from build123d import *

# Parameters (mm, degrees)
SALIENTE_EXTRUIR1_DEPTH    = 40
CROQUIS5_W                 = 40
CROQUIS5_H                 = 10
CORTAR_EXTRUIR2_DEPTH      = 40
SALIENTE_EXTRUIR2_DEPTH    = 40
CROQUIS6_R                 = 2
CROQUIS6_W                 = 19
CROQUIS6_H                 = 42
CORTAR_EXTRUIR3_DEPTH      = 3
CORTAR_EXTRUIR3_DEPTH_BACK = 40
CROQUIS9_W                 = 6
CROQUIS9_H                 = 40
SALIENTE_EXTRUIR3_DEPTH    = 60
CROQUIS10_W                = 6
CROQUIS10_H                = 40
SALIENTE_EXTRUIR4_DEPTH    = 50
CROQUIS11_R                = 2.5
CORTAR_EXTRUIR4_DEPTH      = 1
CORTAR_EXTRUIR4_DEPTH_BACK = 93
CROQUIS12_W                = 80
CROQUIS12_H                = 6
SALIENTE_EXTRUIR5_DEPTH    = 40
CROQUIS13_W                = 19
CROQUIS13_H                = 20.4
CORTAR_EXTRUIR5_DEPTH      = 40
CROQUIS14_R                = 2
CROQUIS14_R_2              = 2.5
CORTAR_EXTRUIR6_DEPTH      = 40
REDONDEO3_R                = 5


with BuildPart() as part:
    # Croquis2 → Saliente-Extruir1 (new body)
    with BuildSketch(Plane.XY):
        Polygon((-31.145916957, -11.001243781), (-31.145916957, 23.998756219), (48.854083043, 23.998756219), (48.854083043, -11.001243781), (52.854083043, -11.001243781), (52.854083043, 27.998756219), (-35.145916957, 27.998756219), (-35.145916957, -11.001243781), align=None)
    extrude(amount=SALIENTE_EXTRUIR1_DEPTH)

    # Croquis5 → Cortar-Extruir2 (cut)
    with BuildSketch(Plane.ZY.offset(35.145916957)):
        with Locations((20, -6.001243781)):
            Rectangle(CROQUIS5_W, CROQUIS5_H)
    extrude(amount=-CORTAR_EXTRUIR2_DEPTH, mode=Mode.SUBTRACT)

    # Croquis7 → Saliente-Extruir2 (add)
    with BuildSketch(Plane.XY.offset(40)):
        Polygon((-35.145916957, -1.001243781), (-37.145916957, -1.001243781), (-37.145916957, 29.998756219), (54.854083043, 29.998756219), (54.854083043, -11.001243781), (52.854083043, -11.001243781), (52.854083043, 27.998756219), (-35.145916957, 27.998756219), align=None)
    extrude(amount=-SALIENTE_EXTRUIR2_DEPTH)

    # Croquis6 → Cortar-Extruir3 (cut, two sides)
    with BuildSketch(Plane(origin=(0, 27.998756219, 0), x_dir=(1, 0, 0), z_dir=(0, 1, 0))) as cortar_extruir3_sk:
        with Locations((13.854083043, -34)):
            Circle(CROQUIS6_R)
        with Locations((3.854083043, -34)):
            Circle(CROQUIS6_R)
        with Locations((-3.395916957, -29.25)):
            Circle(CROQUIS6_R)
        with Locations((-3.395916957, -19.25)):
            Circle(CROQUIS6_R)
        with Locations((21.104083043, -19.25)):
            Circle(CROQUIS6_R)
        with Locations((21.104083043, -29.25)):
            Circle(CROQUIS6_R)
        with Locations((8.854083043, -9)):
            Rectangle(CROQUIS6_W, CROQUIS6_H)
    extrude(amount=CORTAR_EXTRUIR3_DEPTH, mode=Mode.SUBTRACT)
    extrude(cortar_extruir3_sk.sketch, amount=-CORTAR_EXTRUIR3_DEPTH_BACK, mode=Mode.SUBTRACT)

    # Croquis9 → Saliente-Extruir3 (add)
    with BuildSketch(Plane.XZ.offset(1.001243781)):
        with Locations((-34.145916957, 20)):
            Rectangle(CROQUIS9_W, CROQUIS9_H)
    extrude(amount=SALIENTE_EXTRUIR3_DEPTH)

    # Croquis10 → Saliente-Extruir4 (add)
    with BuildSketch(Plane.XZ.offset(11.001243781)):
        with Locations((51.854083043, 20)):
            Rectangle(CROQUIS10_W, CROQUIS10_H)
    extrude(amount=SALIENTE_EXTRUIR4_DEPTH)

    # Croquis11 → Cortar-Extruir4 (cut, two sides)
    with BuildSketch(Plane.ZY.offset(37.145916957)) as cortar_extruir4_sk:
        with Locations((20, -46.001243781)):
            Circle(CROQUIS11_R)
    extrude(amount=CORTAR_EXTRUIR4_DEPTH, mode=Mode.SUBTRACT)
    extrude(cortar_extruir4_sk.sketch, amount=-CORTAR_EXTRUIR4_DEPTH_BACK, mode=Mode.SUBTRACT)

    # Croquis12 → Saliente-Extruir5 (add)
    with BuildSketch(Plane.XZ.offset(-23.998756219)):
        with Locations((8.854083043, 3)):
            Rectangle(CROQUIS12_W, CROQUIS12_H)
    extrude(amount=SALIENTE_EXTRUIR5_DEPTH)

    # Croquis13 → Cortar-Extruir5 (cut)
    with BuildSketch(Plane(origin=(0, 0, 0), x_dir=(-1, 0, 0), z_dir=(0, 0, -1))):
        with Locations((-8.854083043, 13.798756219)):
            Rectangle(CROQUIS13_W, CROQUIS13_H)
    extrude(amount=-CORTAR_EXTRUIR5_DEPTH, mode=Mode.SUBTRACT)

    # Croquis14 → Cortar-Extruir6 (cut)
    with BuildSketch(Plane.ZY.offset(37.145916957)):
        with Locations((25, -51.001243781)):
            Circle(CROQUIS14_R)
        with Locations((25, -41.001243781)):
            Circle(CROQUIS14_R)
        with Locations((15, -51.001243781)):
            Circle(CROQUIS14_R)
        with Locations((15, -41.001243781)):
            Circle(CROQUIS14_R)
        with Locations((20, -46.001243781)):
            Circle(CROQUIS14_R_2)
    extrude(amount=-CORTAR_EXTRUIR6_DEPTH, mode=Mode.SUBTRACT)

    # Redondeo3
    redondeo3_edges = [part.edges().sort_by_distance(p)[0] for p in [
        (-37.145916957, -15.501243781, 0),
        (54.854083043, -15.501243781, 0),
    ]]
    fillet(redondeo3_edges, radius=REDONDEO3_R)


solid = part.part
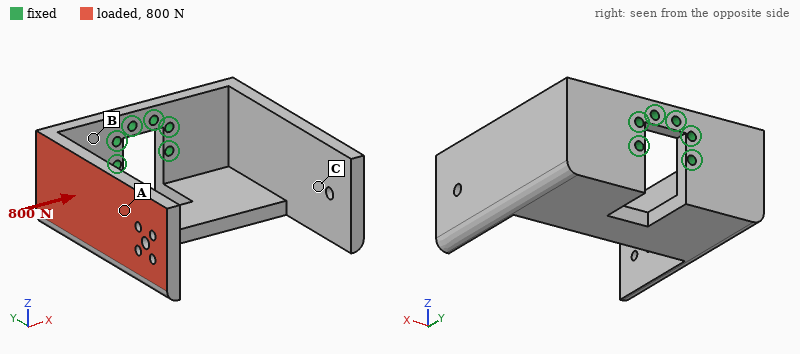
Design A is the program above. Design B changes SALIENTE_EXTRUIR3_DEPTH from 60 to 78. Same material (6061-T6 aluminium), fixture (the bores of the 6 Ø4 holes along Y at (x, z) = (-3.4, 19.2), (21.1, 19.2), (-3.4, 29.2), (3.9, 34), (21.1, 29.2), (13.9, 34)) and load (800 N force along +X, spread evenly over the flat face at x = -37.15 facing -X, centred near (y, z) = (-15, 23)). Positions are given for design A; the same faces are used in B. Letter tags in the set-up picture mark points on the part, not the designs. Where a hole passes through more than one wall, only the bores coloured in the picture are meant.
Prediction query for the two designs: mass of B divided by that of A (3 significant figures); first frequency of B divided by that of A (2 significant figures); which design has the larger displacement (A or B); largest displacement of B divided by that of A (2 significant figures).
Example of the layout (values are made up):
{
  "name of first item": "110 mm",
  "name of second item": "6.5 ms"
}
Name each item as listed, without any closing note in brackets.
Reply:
{
  "mass of B divided by that of A": "1.06",
  "first frequency of B divided by that of A": "0.80",
  "which design has the larger displacement": "B",
  "largest displacement of B divided by that of A": "1.8"
}
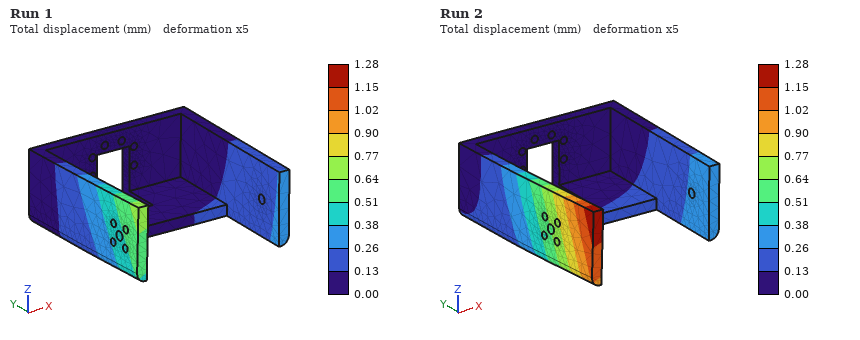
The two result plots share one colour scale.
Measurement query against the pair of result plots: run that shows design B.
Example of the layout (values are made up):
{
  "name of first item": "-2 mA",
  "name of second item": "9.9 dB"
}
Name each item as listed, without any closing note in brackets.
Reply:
{
  "run that shows design B": "Run 2"
}
